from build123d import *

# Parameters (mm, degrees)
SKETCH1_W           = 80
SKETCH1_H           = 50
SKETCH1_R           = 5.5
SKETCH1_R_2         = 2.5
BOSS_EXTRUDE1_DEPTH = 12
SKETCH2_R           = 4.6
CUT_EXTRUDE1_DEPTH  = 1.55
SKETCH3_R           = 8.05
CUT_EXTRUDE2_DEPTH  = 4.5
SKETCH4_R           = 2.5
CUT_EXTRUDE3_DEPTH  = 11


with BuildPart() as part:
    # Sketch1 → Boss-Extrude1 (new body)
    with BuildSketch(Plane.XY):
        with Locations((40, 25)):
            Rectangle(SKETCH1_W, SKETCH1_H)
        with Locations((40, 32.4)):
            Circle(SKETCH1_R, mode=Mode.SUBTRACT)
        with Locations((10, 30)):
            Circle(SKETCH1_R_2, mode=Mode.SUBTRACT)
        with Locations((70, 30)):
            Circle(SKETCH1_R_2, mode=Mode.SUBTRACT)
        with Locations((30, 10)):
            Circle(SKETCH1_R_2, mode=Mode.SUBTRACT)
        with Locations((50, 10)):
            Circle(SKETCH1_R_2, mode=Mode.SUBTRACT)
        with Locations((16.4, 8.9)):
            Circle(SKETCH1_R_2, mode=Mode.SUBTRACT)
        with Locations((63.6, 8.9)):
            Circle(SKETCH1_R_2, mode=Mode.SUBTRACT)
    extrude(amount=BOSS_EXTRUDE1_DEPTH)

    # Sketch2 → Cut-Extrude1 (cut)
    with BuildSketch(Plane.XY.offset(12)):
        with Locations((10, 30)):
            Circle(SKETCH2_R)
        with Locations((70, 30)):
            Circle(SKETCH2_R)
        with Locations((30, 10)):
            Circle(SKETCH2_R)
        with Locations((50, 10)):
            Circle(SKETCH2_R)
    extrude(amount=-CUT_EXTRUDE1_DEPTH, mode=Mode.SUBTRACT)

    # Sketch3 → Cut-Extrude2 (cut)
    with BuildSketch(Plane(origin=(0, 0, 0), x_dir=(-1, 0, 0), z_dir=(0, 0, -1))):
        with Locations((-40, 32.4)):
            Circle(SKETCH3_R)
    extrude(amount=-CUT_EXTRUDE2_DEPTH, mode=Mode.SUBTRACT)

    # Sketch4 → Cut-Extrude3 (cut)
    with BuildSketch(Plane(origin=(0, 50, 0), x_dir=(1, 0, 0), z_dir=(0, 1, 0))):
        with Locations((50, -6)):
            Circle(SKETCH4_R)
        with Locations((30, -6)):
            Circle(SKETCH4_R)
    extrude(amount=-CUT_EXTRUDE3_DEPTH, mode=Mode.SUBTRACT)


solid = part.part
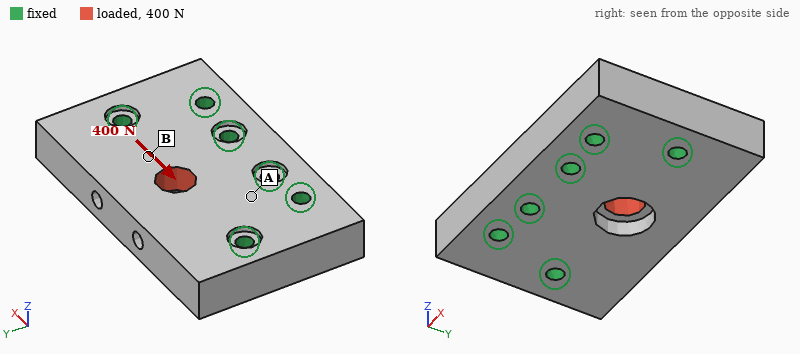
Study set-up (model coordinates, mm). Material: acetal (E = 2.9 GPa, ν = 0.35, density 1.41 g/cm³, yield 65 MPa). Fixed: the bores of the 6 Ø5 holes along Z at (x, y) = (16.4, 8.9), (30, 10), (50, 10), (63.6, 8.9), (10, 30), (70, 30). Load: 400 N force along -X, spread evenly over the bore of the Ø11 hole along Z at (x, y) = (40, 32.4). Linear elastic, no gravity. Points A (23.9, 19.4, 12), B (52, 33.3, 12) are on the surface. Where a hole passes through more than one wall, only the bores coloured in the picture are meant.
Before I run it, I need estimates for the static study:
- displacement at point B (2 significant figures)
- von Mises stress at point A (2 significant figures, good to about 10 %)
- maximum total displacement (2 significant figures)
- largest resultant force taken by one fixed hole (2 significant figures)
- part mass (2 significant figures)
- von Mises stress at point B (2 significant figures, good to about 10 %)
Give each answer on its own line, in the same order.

6.5 µm
0.45 MPa
11 µm
140 N
62 g
1.4 MPa
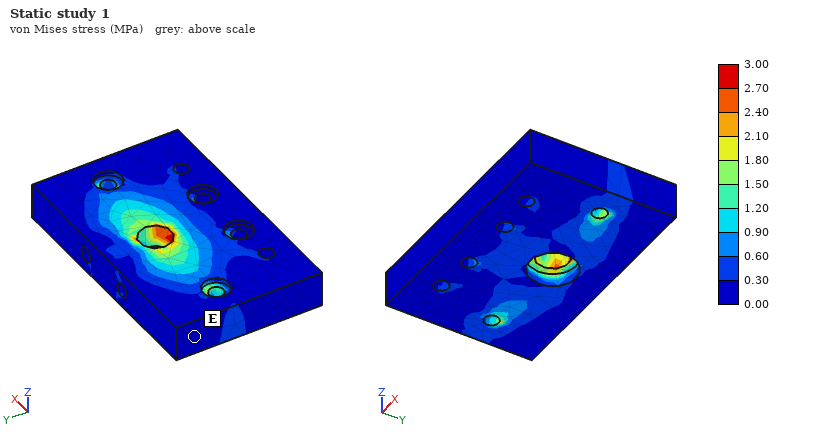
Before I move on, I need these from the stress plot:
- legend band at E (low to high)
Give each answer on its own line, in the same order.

0.00 to 0.30 MPa
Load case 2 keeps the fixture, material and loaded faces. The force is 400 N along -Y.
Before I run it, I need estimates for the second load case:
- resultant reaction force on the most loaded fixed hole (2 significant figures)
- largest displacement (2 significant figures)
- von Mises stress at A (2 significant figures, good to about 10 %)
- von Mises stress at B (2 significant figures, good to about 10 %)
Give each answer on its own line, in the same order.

130 N
17 µm
0.74 MPa
0.76 MPa
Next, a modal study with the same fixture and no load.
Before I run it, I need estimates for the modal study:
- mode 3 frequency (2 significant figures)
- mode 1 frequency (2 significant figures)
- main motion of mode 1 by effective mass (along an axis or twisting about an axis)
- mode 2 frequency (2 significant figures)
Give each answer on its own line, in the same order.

6200 Hz
3300 Hz
along Z
5200 Hz
